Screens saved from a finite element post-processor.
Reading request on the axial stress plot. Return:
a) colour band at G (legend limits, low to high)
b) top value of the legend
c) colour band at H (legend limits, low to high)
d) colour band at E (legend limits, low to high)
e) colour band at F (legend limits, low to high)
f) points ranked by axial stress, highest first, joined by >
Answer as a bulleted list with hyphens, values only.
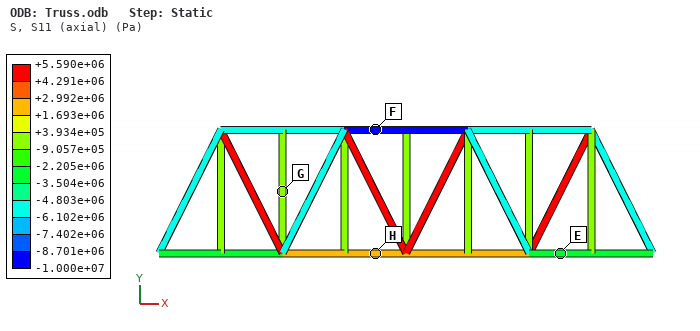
- -9.057e+05 to +3.934e+05 Pa
- +5.590e+06 Pa
- +1.693e+06 to +2.992e+06 Pa
- -3.504e+06 to -2.205e+06 Pa
- -1.000e+07 to -8.701e+06 Pa
- H > G > E > F
